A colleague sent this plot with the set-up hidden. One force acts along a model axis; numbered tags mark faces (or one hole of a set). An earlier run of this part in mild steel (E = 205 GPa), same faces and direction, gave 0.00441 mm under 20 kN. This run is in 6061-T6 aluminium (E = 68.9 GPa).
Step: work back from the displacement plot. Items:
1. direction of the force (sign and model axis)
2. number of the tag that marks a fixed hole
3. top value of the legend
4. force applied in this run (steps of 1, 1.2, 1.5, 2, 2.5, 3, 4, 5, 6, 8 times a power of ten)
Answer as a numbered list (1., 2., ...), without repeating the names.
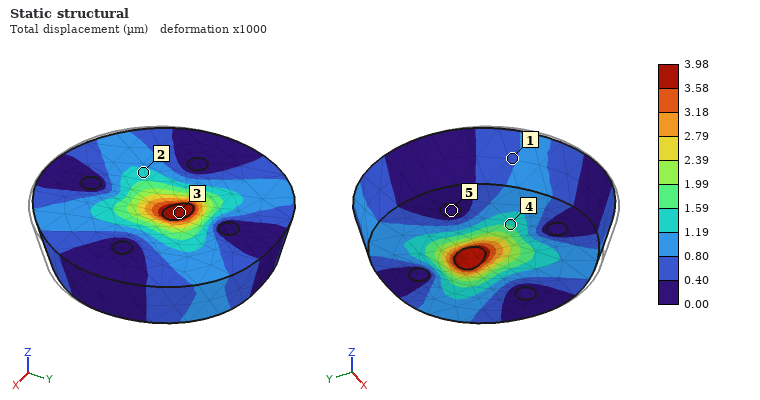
1. +Y
2. 5
3. 3.98 µm
4. 6 kN
